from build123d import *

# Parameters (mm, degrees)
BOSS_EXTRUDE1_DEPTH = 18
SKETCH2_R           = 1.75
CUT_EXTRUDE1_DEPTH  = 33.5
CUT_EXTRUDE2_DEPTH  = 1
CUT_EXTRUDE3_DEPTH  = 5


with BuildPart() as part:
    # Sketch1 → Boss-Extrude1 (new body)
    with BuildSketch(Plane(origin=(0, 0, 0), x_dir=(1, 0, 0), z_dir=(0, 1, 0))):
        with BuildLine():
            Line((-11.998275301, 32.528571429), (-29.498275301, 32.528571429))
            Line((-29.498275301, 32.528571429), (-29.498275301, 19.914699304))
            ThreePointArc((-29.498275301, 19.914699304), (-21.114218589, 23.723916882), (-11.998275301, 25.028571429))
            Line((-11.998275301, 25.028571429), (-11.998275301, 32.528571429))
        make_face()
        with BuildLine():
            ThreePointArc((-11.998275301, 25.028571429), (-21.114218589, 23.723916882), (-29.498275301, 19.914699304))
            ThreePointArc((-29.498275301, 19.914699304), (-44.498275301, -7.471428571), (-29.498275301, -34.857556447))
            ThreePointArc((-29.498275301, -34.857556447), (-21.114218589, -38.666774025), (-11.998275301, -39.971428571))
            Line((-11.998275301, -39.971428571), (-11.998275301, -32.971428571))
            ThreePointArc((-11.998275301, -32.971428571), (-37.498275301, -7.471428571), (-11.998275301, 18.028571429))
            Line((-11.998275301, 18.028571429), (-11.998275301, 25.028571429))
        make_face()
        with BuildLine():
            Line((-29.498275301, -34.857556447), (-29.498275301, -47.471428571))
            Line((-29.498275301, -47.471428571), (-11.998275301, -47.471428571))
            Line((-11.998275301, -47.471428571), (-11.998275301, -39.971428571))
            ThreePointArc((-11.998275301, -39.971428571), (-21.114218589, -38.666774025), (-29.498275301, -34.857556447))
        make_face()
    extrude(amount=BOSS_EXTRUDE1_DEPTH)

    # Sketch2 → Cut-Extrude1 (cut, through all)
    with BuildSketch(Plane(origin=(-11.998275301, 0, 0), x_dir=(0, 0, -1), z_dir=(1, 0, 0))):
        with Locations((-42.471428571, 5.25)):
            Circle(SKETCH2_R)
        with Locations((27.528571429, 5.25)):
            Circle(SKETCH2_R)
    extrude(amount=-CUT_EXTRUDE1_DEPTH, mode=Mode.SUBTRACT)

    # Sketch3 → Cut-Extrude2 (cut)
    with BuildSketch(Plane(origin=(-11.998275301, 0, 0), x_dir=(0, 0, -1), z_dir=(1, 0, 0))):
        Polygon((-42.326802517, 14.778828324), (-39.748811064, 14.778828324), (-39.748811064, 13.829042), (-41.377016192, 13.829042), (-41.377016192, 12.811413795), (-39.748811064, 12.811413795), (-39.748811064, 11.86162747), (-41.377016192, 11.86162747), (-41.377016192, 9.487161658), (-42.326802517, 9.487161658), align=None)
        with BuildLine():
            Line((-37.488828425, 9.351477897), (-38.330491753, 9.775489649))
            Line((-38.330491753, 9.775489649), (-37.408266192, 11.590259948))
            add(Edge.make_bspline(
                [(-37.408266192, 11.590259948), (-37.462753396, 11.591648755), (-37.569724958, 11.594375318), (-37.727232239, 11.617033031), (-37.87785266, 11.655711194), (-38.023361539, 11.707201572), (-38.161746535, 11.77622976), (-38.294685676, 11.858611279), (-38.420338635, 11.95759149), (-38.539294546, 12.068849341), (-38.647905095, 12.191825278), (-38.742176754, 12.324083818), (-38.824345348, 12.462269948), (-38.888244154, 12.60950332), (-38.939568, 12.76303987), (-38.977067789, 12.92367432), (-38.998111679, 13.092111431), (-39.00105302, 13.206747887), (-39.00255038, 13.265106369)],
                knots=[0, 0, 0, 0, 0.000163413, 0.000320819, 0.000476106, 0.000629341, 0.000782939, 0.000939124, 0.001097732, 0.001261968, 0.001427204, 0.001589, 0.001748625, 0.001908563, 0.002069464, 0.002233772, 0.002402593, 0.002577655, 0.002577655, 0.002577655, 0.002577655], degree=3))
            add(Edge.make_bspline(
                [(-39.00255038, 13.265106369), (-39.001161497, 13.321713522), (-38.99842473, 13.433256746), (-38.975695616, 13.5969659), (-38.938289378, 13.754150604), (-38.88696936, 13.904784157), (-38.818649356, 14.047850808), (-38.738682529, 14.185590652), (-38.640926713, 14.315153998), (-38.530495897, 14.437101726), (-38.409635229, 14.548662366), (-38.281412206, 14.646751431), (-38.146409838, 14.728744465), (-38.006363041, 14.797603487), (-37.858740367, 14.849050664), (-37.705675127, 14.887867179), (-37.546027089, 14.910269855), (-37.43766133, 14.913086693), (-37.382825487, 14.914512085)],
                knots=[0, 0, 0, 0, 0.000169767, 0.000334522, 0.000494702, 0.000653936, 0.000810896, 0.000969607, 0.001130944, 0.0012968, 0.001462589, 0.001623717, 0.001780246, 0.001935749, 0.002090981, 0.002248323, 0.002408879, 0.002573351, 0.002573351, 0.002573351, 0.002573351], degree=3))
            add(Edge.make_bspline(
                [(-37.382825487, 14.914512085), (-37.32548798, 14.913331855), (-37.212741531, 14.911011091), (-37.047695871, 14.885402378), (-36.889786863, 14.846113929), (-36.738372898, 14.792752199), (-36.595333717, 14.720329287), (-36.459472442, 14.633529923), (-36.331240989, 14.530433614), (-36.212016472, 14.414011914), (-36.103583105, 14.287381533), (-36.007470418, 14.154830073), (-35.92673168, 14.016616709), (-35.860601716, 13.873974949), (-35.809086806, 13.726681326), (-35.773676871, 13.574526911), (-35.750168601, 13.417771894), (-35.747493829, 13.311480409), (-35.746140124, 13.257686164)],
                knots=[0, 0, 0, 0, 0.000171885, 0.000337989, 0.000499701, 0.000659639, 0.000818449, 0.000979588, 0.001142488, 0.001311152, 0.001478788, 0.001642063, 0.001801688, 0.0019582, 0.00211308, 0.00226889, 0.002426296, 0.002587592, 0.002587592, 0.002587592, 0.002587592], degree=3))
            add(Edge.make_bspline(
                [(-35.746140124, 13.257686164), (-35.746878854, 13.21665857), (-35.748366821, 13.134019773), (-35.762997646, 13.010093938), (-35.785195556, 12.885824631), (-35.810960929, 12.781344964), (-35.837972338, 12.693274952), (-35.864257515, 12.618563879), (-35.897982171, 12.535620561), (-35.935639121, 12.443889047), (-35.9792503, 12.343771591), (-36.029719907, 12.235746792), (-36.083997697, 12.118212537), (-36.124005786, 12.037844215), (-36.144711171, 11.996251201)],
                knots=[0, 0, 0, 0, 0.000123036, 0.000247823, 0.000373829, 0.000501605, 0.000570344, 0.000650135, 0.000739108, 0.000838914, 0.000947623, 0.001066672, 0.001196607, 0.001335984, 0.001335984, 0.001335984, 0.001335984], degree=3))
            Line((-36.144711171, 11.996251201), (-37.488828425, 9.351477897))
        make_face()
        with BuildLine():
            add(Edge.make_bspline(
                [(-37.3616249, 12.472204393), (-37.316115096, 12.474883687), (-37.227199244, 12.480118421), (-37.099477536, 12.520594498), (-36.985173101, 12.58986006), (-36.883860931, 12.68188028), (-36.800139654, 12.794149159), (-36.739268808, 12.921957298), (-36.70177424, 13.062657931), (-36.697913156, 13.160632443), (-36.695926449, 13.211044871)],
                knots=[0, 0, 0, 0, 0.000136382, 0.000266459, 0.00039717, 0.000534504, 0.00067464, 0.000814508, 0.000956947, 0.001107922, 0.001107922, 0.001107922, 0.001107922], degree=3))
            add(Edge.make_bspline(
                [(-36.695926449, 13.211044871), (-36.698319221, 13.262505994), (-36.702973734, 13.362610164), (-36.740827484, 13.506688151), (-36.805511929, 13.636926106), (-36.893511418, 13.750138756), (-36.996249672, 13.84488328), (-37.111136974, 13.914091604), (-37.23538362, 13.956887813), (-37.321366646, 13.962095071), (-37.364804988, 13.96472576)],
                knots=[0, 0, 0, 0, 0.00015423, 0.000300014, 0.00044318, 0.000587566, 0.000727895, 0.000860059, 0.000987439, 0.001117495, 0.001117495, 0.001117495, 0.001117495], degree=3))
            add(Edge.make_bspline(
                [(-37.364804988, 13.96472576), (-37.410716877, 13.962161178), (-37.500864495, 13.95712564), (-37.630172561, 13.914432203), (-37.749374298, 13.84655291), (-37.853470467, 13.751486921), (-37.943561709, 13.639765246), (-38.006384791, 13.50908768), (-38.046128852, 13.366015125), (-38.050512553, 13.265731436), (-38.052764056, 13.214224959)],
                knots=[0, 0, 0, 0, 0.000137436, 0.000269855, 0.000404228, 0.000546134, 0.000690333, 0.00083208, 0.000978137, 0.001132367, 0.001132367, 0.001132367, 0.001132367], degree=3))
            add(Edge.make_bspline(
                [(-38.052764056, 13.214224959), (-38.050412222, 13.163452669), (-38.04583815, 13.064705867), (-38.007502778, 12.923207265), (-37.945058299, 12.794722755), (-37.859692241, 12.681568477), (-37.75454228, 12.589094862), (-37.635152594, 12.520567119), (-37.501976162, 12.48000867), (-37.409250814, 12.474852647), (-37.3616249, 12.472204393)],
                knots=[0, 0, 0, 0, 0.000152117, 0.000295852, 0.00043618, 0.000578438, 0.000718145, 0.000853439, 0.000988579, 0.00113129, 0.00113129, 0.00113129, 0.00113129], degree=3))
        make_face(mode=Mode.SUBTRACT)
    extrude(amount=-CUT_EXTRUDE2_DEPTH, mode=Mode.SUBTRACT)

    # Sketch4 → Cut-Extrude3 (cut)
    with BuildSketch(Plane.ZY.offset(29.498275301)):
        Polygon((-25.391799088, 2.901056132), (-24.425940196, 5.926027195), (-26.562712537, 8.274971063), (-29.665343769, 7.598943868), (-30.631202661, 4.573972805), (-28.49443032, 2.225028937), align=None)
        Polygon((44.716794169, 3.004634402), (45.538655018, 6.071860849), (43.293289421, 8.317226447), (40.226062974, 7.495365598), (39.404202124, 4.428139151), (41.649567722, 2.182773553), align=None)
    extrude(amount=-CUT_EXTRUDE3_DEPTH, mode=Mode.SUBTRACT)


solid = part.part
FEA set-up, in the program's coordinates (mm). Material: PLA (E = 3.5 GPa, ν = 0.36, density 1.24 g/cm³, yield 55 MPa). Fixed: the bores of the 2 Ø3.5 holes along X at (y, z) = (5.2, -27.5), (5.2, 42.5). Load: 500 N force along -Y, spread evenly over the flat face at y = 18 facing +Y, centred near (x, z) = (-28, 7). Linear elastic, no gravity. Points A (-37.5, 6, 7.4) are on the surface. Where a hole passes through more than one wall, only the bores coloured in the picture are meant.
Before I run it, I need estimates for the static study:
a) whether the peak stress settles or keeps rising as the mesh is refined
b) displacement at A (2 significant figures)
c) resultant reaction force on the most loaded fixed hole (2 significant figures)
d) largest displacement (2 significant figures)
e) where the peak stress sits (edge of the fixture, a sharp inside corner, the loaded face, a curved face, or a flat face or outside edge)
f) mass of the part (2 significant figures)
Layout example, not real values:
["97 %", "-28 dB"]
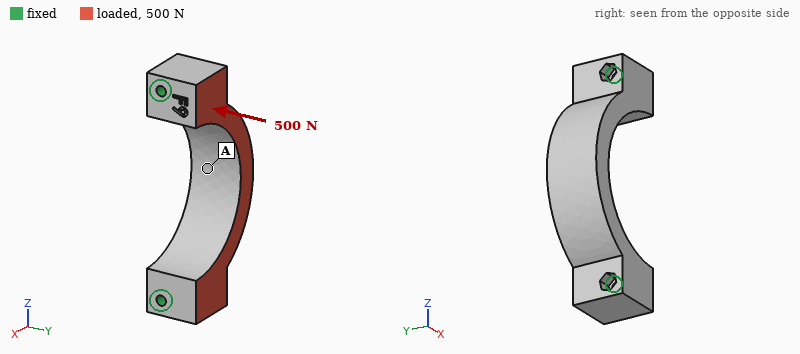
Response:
["keeps rising", "0.13 mm", "250 N", "0.19 mm", "edge of the fixture", "21 g"]
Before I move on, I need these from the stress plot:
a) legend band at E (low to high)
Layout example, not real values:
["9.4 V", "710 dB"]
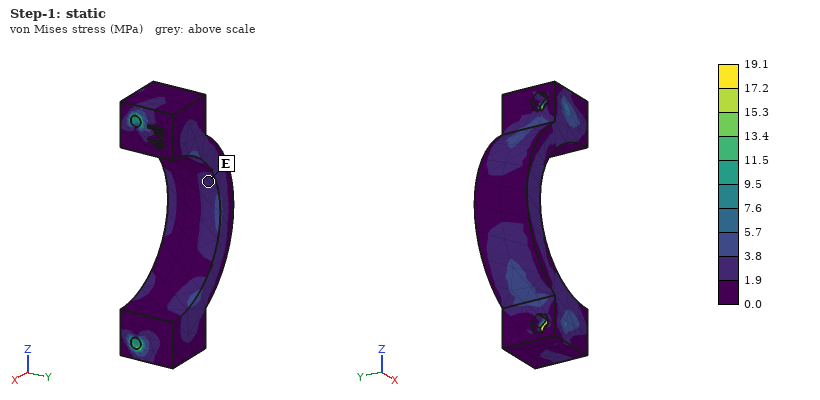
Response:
["1.9 to 3.8 MPa"]
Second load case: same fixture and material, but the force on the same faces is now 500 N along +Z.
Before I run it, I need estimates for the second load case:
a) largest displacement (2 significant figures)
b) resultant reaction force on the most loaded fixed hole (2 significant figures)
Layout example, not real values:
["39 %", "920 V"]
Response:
["55 µm", "260 N"]
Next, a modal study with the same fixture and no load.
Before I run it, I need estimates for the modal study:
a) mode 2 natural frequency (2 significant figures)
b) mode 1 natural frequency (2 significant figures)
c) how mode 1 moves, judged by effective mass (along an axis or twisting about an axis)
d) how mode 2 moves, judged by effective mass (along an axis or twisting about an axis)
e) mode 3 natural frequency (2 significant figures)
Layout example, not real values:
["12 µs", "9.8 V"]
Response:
["4200 Hz", "2200 Hz", "along Y", "along Z", "5700 Hz"]
